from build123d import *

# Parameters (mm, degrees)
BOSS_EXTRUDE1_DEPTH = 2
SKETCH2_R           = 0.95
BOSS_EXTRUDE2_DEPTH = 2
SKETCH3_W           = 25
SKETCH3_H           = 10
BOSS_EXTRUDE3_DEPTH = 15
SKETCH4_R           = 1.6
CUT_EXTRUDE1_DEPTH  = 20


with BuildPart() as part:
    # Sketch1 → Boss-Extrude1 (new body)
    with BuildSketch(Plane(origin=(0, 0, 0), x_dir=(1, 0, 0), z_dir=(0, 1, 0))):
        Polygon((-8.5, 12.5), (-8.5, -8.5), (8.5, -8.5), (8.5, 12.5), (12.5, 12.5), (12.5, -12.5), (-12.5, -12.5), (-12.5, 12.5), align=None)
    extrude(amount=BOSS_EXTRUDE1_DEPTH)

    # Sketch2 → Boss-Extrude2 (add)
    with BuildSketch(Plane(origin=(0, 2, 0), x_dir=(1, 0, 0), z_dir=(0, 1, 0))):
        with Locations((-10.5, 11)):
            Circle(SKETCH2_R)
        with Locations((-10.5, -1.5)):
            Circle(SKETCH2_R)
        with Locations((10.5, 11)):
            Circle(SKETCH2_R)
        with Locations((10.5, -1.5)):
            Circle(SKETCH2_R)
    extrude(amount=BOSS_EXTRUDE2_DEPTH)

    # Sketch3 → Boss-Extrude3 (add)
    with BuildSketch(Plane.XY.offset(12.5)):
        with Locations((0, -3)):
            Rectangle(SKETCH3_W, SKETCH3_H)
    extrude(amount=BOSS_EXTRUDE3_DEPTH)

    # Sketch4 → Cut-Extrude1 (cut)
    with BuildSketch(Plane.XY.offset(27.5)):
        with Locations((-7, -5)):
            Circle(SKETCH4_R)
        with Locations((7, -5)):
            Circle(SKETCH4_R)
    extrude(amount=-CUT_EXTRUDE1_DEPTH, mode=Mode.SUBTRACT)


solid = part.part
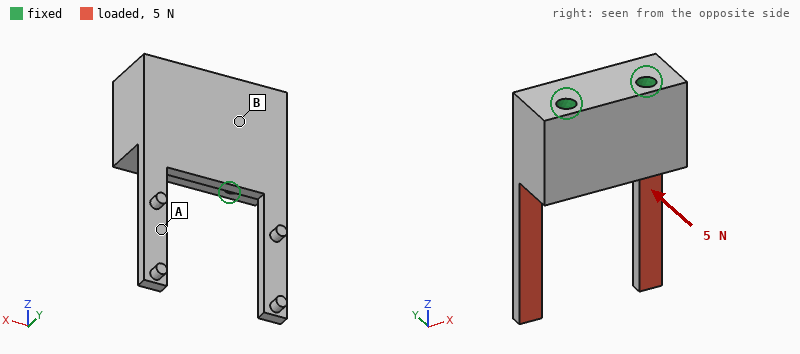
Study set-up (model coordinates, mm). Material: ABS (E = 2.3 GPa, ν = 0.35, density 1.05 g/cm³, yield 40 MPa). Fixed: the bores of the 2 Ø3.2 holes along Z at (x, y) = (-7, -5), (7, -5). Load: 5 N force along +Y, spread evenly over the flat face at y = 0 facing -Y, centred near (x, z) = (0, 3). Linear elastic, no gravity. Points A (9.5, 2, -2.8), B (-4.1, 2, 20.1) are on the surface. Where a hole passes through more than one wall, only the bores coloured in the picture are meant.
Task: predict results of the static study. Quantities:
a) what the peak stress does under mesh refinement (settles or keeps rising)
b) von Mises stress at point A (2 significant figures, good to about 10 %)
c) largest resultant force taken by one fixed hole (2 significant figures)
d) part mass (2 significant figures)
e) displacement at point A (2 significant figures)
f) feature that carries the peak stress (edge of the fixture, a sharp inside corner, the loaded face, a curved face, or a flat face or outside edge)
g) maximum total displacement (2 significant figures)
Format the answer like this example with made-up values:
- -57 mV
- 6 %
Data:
- keeps rising
- 1.3 MPa
- 2.5 N
- 4.3 g
- 0.26 mm
- a sharp inside corner
- 0.55 mm
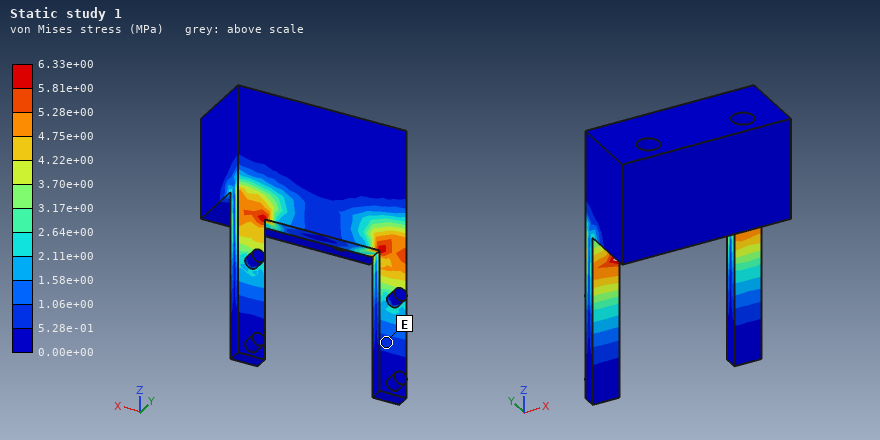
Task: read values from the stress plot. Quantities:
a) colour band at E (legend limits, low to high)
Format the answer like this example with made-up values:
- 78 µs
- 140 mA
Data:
- 5.28e-01 to 1.06e+00 MPa
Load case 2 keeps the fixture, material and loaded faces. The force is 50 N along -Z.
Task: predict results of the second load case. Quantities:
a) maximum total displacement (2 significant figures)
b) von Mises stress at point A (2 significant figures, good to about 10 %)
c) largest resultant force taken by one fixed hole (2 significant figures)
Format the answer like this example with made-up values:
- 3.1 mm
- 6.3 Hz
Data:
- 0.57 mm
- 1.8 MPa
- 25 N
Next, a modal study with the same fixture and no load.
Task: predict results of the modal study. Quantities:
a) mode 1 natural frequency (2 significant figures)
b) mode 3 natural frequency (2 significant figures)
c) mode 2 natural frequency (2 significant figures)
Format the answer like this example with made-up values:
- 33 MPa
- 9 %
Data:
- 760 Hz
- 1600 Hz
- 760 Hz
